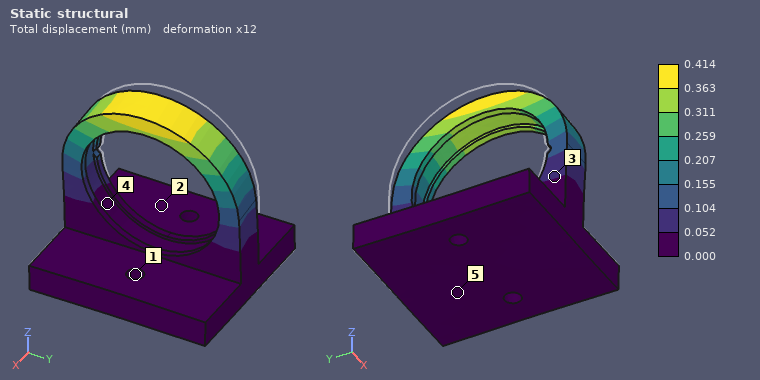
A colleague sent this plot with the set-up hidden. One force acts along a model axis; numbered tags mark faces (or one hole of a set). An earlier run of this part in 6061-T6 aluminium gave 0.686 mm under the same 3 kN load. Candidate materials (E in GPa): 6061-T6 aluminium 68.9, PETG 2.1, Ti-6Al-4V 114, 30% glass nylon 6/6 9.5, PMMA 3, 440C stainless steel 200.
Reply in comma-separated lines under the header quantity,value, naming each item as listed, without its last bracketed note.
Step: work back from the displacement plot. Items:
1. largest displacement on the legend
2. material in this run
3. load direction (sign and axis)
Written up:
quantity,value
largest displacement on the legend,0.414 mm
material in this run,Ti-6Al-4V
load direction,+X
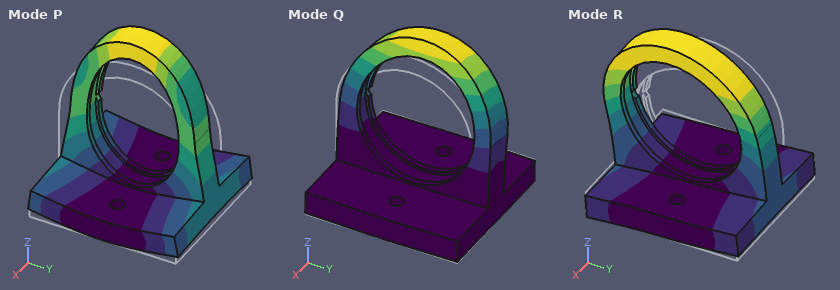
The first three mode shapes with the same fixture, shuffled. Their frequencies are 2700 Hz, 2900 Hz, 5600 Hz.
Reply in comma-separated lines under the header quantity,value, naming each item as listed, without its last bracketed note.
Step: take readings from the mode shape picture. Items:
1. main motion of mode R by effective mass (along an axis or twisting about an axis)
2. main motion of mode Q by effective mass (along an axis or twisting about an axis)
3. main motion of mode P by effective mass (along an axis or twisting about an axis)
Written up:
quantity,value
main motion of mode R by effective mass,along Y
main motion of mode Q by effective mass,along X
main motion of mode P by effective mass,along Z
